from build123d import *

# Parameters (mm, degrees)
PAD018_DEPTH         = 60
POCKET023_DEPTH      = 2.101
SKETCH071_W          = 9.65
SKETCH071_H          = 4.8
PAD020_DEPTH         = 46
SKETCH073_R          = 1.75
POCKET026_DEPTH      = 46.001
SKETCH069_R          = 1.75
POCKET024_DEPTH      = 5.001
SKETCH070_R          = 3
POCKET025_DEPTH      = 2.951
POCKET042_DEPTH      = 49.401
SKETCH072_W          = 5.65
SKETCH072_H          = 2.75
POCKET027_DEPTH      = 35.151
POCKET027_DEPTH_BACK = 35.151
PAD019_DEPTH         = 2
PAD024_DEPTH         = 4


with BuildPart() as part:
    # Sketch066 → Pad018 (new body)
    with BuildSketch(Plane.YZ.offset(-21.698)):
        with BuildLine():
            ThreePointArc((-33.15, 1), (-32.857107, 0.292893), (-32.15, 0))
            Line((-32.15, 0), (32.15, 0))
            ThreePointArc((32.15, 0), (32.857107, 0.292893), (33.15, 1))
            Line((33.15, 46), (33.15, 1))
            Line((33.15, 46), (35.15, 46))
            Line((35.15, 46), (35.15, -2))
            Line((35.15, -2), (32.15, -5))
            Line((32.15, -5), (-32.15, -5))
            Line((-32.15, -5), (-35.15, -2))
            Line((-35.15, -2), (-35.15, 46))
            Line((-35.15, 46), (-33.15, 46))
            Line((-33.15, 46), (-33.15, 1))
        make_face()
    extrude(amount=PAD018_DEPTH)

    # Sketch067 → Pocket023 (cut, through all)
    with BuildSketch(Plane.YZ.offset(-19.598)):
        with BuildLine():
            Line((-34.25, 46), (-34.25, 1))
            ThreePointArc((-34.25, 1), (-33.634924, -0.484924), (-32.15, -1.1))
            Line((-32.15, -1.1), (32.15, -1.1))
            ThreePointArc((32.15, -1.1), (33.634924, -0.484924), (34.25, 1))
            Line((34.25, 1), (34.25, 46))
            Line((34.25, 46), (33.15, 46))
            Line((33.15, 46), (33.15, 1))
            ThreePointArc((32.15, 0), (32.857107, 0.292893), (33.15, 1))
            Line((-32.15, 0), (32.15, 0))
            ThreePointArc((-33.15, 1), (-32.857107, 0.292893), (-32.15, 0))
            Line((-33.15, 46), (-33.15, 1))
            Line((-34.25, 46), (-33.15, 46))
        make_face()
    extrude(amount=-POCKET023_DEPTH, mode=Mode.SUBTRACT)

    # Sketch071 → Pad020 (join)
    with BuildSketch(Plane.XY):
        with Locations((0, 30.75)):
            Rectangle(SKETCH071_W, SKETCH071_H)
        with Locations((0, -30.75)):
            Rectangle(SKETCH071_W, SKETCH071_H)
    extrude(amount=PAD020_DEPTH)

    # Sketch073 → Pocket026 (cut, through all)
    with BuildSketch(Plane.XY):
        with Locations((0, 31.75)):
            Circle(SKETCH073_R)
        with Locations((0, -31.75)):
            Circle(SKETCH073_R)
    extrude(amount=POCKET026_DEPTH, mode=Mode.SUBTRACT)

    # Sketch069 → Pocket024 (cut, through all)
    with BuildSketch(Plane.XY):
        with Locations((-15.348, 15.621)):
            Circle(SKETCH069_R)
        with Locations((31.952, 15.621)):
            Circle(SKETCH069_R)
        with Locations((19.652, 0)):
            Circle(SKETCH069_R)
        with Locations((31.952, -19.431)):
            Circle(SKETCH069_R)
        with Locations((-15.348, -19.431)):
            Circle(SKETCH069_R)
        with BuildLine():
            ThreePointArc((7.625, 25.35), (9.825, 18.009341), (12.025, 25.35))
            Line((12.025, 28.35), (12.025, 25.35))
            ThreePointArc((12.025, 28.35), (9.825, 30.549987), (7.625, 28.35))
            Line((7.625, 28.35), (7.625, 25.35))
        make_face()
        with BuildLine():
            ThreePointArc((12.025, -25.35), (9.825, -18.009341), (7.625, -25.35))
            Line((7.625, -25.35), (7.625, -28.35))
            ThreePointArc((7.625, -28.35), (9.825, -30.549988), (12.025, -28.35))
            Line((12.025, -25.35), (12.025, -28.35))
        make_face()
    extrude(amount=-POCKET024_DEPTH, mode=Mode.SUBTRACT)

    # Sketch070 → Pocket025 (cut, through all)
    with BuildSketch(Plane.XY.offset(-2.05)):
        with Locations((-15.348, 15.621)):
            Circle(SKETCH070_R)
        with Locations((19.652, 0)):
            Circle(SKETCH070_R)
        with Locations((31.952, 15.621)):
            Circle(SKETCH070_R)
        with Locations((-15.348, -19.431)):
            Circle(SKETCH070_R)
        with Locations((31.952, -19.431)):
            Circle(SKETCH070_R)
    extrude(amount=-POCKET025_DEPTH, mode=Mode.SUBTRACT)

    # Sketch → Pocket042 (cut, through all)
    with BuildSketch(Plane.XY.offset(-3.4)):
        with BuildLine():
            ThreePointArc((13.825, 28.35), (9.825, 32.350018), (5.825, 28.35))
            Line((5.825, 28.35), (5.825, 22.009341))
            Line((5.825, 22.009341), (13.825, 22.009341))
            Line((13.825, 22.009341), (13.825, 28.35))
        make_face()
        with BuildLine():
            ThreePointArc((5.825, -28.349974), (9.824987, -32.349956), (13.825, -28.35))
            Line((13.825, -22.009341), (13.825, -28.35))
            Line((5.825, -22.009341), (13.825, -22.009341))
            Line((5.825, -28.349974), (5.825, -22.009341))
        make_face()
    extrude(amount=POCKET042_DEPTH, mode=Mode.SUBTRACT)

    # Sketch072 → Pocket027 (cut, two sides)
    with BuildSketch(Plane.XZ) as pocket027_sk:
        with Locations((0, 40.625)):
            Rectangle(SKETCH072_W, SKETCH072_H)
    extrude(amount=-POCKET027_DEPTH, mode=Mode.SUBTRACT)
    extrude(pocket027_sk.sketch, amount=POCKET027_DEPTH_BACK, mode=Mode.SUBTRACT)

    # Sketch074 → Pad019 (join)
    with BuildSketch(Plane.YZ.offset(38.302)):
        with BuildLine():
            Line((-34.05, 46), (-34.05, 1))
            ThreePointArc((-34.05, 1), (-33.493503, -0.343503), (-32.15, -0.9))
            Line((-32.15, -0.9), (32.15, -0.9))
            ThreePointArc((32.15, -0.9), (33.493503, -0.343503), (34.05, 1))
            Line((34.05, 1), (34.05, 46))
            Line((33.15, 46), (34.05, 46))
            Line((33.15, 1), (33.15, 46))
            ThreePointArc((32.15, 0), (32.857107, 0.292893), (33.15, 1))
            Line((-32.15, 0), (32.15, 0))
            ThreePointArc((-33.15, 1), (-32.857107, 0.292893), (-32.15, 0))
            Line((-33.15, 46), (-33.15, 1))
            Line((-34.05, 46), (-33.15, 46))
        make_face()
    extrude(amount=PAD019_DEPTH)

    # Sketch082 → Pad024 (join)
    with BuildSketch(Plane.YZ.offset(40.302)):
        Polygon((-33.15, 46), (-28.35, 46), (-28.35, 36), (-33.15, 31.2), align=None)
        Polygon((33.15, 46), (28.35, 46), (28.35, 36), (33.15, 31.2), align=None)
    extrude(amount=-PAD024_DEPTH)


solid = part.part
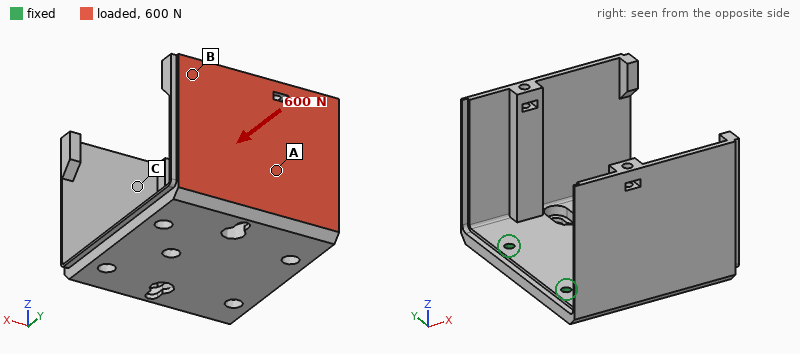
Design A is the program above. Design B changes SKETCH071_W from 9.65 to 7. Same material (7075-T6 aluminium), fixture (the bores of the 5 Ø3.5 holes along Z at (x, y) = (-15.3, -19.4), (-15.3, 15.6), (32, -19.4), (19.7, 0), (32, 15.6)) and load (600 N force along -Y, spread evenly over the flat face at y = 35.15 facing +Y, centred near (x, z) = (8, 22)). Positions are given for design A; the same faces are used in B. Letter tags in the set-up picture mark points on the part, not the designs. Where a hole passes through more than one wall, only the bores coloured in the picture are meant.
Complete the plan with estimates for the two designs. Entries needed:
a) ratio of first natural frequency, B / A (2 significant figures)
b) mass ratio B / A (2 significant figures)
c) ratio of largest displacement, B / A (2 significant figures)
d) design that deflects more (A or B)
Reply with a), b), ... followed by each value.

a) 0.98
b) 0.97
c) 1.1
d) B
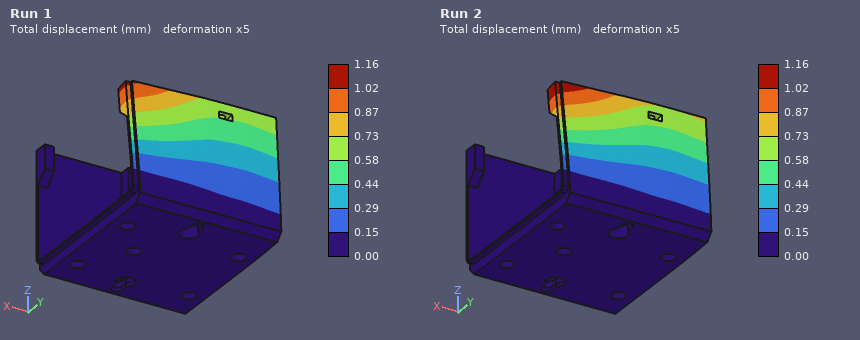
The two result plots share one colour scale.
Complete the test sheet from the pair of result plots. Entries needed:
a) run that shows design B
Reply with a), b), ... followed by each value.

a) Run 2
